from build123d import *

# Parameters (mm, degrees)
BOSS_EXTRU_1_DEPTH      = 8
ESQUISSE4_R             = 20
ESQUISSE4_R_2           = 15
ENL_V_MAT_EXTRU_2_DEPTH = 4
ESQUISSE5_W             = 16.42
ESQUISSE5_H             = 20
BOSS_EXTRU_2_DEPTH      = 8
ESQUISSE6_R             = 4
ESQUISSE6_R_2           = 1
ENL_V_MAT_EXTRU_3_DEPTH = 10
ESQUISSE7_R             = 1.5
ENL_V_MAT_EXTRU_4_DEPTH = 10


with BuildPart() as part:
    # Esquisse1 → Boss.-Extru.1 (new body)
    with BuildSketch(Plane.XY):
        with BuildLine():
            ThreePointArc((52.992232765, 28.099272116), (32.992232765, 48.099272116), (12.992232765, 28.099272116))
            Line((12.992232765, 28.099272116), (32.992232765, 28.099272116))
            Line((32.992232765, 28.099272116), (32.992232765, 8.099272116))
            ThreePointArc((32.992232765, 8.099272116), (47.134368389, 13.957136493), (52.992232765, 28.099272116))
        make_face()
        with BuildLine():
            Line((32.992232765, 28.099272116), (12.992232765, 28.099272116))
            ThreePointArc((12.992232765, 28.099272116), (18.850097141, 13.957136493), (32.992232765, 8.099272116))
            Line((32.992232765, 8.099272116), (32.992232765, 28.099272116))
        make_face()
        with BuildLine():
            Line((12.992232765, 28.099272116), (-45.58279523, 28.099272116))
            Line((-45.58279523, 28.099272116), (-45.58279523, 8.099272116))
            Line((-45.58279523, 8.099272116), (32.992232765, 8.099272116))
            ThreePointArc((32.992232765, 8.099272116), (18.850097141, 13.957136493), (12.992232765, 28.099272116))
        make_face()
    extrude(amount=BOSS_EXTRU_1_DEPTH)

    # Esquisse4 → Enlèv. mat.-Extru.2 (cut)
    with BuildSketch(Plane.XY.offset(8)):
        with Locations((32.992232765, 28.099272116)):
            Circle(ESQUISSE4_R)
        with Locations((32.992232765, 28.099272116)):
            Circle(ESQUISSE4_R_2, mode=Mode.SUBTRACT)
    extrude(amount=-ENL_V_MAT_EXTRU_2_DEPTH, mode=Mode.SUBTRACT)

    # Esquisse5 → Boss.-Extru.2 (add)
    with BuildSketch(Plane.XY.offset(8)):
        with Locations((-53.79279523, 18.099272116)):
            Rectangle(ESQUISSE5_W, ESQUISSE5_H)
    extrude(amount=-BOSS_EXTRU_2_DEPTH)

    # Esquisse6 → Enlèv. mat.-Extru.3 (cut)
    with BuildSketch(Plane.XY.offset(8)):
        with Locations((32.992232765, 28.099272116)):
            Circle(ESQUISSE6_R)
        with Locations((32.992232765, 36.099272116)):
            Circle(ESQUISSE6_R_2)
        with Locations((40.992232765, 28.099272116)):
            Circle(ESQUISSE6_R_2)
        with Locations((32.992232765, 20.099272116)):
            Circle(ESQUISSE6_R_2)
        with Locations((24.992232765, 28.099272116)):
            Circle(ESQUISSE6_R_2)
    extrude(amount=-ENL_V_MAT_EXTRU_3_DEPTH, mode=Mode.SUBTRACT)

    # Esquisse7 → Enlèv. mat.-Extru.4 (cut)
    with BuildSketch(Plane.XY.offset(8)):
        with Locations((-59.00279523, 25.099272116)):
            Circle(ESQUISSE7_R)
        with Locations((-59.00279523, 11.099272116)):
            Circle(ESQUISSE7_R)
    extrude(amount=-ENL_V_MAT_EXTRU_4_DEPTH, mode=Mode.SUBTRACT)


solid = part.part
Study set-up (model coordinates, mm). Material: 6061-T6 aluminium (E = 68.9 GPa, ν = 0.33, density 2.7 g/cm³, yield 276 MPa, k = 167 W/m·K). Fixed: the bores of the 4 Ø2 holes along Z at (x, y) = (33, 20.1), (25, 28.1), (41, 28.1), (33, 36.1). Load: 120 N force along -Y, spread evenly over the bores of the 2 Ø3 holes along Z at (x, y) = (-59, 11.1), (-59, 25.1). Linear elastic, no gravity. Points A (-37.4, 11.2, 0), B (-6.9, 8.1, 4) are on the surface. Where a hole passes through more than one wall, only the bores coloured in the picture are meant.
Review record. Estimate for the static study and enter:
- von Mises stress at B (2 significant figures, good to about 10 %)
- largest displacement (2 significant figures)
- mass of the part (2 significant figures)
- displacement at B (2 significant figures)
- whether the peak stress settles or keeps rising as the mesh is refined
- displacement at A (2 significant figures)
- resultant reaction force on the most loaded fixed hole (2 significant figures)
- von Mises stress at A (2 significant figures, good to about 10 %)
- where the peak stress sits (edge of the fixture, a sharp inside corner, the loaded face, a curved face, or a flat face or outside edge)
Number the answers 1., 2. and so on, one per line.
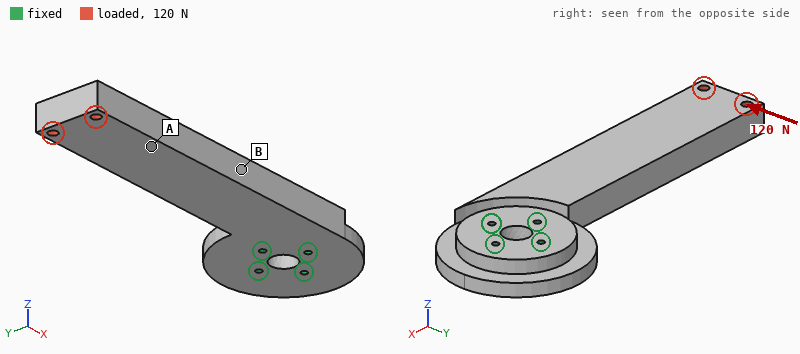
1. 12 MPa
2. 94 µm
3. 54 g
4. 23 µm
5. keeps rising
6. 59 µm
7. 490 N
8. 3.5 MPa
9. a sharp inside corner
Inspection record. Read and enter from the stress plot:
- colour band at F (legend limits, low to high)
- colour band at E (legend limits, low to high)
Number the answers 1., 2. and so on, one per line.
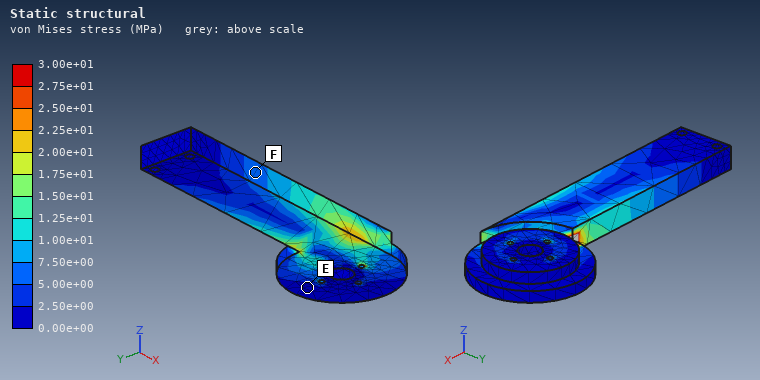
1. 5.00e+00 to 7.50e+00 MPa
2. 0.00e+00 to 2.50e+00 MPa
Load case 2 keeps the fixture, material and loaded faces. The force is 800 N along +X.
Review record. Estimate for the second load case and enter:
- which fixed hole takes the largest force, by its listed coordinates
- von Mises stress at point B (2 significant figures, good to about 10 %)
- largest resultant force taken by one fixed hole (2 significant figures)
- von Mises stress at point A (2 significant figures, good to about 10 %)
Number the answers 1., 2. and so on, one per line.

1. (33, 20.1)
2. 5.0 MPa
3. 550 N
4. 5.0 MPa
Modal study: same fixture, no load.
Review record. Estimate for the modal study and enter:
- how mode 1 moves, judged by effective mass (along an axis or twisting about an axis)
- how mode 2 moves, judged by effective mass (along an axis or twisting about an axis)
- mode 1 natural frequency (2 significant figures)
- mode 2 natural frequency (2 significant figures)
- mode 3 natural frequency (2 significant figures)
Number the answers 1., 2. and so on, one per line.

1. along Z
2. along Y
3. 570 Hz
4. 1800 Hz
5. 4100 Hz
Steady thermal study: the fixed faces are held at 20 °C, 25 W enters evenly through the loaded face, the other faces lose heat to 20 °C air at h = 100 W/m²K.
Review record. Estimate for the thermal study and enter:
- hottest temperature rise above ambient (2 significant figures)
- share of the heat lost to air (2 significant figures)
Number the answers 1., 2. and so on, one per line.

1. 56 K
2. 55 %
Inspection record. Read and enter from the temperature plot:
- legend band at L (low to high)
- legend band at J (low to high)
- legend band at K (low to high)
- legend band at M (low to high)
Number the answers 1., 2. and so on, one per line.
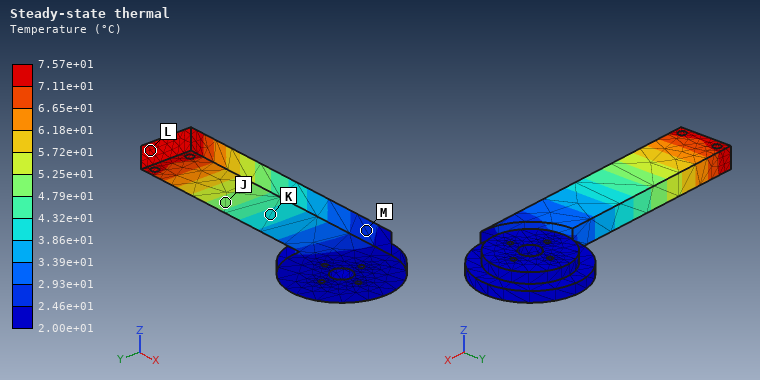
1. 7.11e+01 to 7.57e+01 °C
2. 4.79e+01 to 5.25e+01 °C
3. 3.86e+01 to 4.32e+01 °C
4. 2.46e+01 to 2.93e+01 °C
